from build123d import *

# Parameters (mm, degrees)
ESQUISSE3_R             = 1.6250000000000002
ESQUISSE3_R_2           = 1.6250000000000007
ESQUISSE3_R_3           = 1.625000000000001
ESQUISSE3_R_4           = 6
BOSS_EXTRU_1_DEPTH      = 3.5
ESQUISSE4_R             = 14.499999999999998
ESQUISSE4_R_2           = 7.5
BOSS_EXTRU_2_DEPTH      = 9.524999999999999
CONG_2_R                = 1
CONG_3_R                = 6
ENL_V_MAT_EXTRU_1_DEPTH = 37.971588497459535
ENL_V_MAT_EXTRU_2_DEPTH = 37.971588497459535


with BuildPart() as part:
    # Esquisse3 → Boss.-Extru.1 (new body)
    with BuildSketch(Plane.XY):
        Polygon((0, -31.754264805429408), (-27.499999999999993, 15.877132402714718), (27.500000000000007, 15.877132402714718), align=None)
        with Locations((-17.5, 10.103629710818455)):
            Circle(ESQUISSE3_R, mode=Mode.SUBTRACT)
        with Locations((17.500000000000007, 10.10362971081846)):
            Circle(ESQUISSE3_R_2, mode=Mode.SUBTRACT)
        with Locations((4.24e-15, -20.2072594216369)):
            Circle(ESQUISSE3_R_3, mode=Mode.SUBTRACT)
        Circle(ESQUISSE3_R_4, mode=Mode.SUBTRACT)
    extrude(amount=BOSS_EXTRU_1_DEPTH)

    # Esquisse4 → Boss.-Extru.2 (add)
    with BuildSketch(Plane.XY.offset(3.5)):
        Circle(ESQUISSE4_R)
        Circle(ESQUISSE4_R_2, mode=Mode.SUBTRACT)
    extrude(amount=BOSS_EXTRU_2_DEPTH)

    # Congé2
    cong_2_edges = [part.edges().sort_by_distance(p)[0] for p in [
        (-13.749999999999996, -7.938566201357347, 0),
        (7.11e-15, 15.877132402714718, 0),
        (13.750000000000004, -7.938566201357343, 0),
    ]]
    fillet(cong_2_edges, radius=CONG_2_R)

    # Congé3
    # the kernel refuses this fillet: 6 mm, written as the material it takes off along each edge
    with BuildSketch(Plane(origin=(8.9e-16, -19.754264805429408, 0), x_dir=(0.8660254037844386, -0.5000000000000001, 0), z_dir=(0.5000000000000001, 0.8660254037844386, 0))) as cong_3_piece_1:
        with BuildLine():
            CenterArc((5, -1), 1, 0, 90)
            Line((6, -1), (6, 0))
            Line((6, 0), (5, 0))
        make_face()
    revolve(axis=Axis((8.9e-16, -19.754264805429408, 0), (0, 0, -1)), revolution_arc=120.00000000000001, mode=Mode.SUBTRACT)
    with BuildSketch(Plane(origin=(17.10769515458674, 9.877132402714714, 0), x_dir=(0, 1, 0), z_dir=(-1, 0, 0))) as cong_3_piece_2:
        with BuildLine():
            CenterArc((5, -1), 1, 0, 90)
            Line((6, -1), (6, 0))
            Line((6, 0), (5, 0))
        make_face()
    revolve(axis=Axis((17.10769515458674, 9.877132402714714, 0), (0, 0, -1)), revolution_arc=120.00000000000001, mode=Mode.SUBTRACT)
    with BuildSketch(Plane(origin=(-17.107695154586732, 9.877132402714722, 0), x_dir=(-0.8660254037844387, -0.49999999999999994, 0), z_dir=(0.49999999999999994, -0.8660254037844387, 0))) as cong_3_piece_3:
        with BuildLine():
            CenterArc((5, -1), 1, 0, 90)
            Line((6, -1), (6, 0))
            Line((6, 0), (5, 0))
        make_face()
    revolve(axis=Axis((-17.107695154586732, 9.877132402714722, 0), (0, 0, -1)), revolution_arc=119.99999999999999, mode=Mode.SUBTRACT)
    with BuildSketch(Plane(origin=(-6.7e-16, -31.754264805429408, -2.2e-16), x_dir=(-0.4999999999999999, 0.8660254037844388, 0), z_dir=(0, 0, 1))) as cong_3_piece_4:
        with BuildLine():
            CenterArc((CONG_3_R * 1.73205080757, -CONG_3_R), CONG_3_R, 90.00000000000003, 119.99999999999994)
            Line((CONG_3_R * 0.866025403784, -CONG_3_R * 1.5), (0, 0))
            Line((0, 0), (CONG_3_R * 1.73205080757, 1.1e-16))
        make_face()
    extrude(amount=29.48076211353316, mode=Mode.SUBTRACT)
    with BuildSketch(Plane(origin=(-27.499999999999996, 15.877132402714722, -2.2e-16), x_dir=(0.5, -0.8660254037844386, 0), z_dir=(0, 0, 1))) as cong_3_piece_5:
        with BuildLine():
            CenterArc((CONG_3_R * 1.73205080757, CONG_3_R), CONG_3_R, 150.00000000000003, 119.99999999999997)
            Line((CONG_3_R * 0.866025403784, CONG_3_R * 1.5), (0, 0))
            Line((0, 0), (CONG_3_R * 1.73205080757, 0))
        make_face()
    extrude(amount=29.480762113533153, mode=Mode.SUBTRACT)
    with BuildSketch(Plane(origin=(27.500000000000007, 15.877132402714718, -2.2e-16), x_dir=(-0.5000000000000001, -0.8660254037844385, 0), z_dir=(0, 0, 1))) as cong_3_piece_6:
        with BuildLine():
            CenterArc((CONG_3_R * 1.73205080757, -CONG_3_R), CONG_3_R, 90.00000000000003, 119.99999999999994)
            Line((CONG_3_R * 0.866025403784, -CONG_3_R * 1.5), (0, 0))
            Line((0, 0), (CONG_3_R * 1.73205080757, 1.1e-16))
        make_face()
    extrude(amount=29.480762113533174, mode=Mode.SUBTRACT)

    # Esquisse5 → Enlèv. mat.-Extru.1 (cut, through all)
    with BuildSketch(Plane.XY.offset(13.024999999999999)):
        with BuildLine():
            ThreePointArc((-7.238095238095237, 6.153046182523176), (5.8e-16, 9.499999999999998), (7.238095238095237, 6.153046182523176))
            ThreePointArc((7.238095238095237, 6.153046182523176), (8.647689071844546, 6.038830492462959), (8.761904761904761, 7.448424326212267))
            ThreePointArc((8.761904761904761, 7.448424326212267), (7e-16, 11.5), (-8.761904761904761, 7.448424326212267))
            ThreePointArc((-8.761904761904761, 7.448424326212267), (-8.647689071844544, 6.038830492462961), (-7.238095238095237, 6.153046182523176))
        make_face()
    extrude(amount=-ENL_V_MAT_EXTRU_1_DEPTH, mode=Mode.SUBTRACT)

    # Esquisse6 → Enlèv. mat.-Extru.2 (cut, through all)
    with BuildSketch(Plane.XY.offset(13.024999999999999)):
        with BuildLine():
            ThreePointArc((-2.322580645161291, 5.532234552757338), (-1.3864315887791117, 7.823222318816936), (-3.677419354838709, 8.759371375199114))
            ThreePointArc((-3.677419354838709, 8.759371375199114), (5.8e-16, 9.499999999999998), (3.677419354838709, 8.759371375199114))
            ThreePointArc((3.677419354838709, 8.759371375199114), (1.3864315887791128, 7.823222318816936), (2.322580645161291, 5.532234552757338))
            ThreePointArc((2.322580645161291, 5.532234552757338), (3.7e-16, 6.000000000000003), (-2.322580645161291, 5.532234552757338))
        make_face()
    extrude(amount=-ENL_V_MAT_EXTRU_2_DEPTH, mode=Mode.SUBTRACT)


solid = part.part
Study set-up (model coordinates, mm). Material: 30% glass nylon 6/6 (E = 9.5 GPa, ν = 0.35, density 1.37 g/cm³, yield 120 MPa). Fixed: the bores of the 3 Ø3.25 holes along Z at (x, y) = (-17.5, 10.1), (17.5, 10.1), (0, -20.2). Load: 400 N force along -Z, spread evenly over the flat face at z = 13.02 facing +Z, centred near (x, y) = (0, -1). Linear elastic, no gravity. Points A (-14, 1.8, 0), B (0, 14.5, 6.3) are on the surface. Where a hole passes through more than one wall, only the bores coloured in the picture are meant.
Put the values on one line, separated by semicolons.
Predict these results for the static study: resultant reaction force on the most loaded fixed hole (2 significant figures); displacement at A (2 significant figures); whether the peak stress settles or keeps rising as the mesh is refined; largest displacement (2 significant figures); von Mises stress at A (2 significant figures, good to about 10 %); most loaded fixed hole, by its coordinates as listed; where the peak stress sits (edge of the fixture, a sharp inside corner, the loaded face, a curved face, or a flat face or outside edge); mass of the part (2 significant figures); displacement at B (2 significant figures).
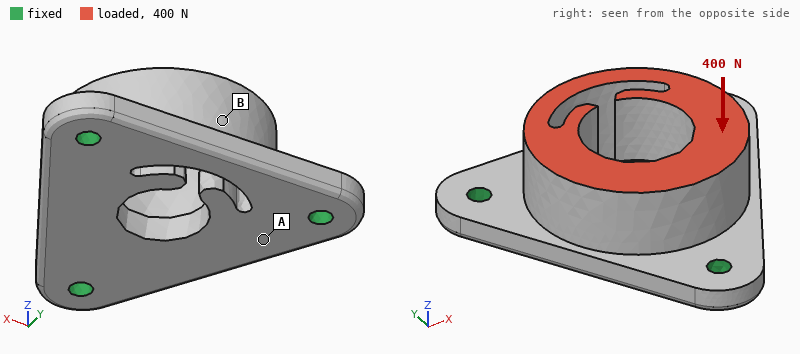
160 N; 17 µm; keeps rising; 25 µm; 4.6 MPa; (0, -20.2); edge of the fixture; 11 g; 22 µm
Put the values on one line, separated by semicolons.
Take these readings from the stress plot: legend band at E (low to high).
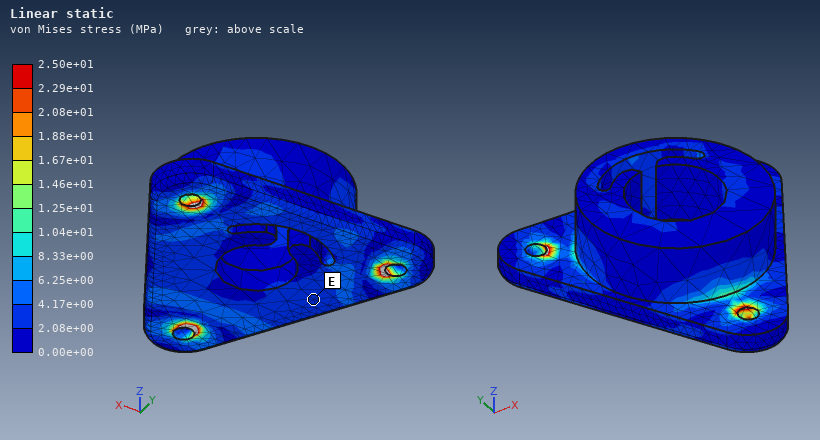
2.08e+00 to 4.17e+00 MPa
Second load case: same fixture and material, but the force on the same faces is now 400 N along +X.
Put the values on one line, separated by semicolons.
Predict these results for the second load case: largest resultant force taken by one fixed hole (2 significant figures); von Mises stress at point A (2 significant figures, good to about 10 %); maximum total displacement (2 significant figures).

210 N; 7.3 MPa; 48 µm
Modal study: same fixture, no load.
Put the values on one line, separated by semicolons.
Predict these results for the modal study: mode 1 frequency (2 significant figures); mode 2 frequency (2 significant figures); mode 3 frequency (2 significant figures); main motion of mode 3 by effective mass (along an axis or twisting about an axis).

7400 Hz; 7600 Hz; 8200 Hz; along Y
